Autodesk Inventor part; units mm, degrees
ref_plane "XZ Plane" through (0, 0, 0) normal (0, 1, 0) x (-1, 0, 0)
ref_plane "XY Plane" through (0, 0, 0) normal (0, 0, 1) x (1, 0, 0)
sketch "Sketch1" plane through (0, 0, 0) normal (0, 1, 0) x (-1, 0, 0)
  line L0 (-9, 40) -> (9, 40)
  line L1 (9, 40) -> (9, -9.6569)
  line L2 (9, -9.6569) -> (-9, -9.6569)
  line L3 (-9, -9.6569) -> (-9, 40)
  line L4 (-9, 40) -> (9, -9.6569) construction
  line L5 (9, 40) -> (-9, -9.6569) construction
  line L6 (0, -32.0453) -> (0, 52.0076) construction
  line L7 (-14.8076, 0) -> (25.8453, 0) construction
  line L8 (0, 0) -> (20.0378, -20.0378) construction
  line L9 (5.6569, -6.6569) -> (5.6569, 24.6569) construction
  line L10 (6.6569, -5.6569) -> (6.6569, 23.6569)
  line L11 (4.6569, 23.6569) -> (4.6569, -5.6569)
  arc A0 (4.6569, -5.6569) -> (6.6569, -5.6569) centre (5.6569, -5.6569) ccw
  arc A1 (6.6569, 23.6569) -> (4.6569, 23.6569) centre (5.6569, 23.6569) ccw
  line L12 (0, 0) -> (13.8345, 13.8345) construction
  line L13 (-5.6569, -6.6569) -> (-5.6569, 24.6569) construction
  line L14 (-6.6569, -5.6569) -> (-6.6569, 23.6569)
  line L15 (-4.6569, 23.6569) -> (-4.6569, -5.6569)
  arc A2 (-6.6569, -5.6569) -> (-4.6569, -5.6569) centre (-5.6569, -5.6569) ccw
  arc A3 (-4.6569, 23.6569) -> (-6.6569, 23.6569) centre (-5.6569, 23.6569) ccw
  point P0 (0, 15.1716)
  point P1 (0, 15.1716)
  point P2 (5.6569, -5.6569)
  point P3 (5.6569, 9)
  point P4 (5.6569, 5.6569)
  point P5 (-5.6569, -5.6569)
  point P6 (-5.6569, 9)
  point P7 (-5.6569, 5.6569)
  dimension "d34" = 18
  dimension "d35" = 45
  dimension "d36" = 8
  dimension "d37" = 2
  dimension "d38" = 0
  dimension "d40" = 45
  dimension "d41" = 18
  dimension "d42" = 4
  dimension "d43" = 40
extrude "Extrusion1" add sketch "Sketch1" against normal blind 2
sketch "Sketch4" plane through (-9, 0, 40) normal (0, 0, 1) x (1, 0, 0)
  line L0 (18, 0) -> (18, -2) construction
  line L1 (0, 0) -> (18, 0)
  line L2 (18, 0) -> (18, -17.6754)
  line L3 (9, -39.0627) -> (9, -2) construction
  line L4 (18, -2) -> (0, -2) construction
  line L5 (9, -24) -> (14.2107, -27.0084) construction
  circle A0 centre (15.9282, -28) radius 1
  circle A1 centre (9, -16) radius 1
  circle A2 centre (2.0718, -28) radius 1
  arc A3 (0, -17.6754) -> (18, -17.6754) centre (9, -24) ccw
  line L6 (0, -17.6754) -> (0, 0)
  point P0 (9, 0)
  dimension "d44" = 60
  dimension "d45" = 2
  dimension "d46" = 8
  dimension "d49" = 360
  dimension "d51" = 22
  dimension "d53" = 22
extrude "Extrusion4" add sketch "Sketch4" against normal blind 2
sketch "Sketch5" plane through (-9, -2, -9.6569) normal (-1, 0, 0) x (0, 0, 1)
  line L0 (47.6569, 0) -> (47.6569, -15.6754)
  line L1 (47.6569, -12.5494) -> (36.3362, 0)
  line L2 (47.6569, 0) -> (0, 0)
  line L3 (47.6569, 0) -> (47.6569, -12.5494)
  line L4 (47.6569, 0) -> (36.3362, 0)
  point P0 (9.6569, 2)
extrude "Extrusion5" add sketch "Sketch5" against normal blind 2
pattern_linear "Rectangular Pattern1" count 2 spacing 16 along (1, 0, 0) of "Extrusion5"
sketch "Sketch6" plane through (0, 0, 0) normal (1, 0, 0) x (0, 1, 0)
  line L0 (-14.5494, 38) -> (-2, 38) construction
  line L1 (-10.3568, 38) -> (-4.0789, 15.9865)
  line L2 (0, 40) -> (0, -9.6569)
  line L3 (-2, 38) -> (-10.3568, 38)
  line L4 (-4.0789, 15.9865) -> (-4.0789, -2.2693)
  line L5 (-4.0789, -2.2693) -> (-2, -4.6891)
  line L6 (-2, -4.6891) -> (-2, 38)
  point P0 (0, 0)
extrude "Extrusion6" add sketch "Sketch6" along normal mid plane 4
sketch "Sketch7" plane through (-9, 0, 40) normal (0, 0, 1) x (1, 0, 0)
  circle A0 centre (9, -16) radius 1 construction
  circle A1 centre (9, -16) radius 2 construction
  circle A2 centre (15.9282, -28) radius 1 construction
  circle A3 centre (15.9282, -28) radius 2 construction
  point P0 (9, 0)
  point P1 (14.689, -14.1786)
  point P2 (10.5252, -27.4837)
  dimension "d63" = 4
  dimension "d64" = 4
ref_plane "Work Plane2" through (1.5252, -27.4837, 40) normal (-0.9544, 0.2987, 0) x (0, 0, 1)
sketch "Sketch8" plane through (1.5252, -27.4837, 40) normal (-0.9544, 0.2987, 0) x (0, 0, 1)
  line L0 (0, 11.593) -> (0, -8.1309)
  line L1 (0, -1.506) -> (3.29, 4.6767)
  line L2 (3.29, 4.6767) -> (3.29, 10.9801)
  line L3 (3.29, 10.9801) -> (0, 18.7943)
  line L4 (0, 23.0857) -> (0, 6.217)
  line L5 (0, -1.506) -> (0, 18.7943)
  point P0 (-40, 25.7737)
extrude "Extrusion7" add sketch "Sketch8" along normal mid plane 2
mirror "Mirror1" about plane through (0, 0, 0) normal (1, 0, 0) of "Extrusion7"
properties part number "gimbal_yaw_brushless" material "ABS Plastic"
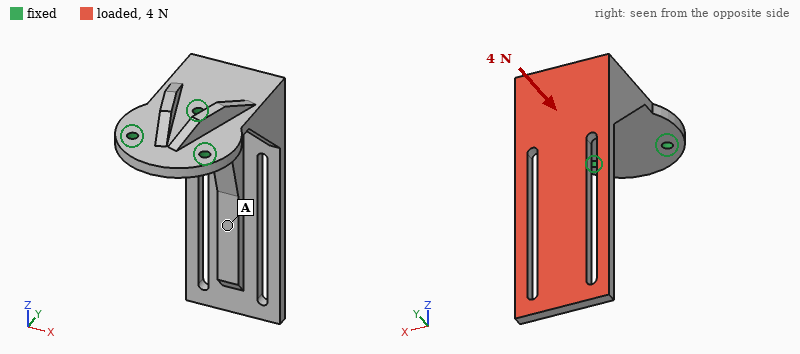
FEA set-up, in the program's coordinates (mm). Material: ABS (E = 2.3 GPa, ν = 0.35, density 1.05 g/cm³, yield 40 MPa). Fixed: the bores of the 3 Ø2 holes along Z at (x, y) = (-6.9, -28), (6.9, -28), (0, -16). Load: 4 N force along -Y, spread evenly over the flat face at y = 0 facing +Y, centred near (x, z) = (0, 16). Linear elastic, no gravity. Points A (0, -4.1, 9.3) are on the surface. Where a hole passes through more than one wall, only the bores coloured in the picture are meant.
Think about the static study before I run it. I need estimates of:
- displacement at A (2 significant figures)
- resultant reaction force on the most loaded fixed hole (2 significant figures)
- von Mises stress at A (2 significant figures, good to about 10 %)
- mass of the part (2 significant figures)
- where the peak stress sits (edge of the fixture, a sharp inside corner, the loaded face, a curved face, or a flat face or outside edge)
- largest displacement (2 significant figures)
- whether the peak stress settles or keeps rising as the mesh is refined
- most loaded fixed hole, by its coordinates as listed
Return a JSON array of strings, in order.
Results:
["0.37 mm", "7.5 N", "1.1 MPa", "4.0 g", "edge of the fixture", "0.68 mm", "keeps rising", "(0, -16)"]
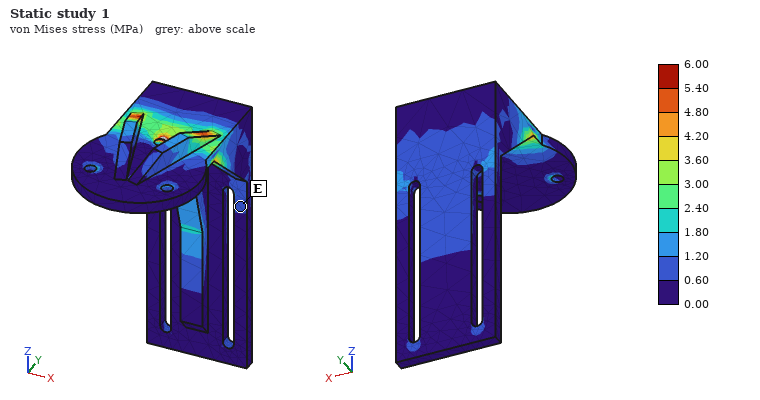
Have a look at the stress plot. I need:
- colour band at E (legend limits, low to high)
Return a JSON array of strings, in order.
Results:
["0.60 to 1.20 MPa"]
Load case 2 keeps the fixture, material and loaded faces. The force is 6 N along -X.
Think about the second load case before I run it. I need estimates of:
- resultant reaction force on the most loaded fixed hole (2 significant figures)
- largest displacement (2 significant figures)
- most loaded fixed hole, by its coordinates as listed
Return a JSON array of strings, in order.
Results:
["12 N", "0.70 mm", "(0, -16)"]
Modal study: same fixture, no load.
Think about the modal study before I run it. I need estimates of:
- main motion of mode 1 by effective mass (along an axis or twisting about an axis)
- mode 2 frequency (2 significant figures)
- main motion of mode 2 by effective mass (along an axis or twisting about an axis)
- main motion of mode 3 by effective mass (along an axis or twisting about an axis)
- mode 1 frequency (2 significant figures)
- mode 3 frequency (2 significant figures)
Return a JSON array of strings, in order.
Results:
["along Y", "400 Hz", "along X", "along Z", "320 Hz", "1400 Hz"]
